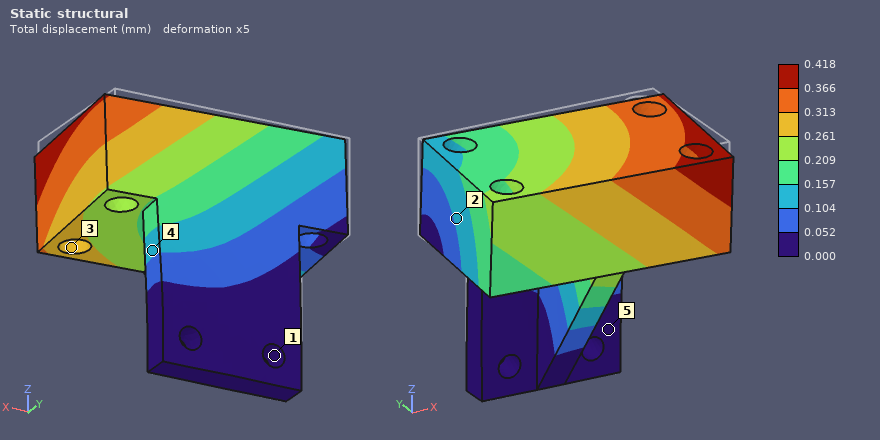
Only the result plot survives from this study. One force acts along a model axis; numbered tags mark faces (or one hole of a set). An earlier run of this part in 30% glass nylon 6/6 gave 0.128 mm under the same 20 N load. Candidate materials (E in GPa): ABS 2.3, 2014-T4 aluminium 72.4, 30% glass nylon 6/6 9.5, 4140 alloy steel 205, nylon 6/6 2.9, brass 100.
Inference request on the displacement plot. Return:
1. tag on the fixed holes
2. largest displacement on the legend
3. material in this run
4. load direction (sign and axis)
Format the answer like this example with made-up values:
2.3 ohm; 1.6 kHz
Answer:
1; 0.418 mm; nylon 6/6; -Y
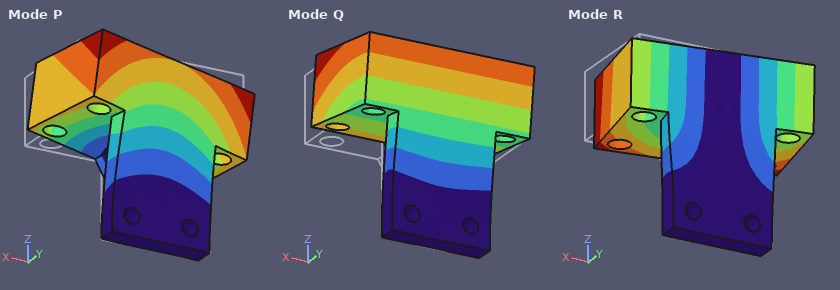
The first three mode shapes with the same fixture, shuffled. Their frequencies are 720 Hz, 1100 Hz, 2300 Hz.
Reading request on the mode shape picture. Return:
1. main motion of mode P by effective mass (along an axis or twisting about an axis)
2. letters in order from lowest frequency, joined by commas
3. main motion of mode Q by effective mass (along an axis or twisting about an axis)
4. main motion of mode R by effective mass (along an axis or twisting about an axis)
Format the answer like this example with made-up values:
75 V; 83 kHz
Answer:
along X; Q, R, P; along Y; along X
